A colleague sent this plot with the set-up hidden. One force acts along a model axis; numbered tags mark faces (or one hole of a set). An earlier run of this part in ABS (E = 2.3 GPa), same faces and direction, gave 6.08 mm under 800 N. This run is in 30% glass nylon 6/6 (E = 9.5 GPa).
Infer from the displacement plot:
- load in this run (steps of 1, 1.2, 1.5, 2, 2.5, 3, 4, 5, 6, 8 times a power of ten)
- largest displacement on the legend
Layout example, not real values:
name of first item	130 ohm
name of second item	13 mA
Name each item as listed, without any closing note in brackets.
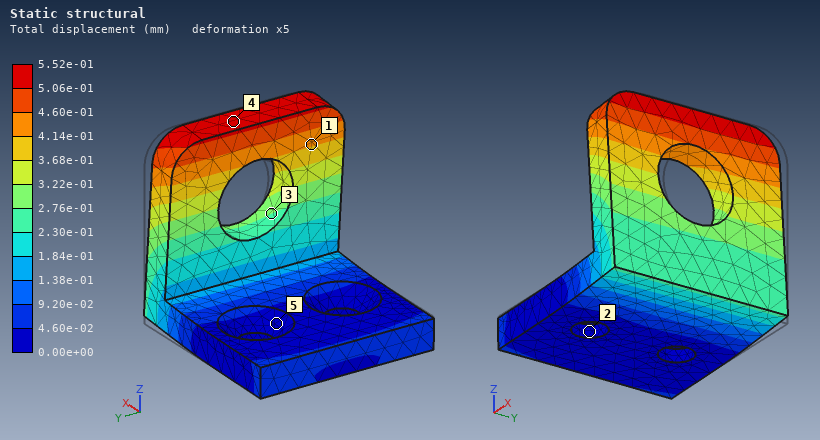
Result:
load in this run	300 N
largest displacement on the legend	5.52e-01 mm
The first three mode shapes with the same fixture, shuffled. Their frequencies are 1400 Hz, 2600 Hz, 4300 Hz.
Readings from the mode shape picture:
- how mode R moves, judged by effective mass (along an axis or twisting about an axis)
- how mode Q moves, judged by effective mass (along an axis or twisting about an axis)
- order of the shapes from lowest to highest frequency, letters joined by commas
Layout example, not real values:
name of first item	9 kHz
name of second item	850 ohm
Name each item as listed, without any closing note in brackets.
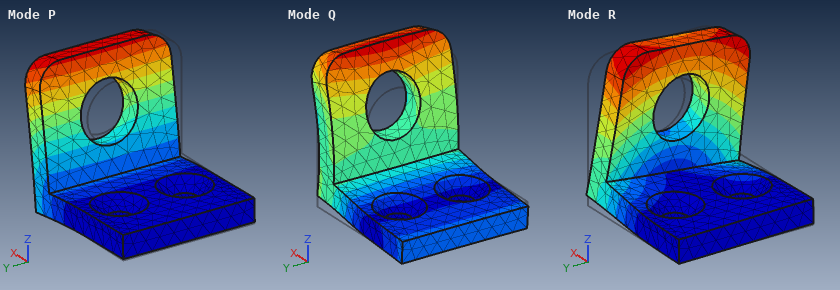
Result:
how mode R moves, judged by effective mass	along Y
how mode Q moves, judged by effective mass	along Z
order of the shapes from lowest to highest frequency, letters joined by commas	P, R, Q
